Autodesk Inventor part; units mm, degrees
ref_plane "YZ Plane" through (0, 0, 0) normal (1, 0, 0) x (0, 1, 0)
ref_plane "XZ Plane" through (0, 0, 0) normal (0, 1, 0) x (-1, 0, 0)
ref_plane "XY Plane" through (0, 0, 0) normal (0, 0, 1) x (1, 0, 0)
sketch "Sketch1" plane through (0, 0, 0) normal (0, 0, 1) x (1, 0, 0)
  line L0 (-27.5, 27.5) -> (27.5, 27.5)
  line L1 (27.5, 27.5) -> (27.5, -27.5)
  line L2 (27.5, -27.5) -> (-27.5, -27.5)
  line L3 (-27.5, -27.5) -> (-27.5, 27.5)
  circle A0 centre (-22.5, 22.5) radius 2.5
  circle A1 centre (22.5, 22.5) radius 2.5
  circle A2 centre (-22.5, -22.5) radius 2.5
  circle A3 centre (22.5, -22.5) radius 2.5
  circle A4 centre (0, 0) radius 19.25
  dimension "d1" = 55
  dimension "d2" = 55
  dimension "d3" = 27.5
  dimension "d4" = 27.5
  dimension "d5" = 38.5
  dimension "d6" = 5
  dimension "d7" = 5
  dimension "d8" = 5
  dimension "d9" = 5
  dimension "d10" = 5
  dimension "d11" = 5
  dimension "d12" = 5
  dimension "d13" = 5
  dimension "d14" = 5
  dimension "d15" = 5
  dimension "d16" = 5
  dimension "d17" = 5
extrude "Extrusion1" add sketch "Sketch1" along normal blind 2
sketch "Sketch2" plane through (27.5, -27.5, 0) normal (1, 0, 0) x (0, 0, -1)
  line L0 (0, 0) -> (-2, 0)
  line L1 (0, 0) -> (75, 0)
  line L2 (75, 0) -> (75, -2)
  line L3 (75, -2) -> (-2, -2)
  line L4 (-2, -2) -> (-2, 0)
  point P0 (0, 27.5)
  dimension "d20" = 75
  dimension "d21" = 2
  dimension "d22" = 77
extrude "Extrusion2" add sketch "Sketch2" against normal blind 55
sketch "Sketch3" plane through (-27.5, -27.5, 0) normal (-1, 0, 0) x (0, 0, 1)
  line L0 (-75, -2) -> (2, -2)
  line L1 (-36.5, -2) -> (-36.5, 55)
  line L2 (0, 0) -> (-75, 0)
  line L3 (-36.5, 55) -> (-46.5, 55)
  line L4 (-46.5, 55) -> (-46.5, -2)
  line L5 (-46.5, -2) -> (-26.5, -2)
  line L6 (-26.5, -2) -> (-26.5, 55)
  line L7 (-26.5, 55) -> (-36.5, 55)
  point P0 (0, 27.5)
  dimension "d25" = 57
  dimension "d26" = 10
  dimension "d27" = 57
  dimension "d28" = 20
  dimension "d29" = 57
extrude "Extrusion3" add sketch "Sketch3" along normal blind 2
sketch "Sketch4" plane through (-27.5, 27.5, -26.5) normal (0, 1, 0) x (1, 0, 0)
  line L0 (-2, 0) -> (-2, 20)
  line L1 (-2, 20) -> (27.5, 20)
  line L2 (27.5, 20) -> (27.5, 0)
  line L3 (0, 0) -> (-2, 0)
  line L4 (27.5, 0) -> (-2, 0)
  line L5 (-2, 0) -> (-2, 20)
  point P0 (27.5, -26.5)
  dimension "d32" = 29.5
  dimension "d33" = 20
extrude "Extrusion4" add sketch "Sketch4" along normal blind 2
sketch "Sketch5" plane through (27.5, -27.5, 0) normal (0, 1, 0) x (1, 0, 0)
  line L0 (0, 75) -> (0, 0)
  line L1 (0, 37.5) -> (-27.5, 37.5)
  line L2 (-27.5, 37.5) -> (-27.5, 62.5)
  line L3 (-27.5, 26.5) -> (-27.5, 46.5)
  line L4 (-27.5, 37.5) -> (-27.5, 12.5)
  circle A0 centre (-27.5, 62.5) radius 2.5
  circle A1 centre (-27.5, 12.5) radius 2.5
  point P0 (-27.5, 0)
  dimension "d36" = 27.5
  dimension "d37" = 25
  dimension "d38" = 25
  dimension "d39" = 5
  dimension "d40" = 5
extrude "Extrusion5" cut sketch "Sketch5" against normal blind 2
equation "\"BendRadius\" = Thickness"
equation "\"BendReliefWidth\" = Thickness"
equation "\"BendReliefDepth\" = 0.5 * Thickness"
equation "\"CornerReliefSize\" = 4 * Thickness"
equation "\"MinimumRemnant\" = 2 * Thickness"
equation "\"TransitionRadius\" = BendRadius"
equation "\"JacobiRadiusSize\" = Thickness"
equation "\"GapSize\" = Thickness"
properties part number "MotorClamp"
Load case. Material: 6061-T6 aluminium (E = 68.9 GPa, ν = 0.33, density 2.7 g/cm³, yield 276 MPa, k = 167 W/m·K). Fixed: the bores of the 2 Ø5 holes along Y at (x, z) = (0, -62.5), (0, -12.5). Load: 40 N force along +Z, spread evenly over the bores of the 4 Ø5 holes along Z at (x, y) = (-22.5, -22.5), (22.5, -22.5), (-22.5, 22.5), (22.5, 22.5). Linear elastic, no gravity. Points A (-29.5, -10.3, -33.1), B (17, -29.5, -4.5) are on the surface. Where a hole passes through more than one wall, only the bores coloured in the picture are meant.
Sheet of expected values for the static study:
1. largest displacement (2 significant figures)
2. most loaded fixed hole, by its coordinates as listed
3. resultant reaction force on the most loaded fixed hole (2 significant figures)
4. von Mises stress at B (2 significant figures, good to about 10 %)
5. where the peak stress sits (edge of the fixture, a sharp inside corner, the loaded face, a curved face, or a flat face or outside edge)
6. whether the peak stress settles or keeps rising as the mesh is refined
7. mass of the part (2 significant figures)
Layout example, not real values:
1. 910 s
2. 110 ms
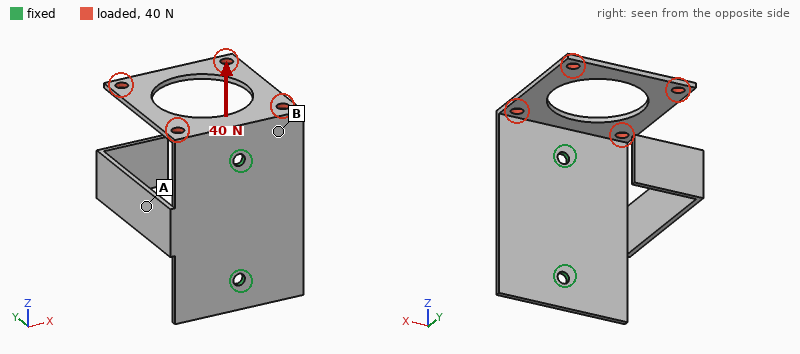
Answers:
1. 1.2 mm
2. (0, -12.5)
3. 26 N
4. 24 MPa
5. edge of the fixture
6. keeps rising
7. 42 g
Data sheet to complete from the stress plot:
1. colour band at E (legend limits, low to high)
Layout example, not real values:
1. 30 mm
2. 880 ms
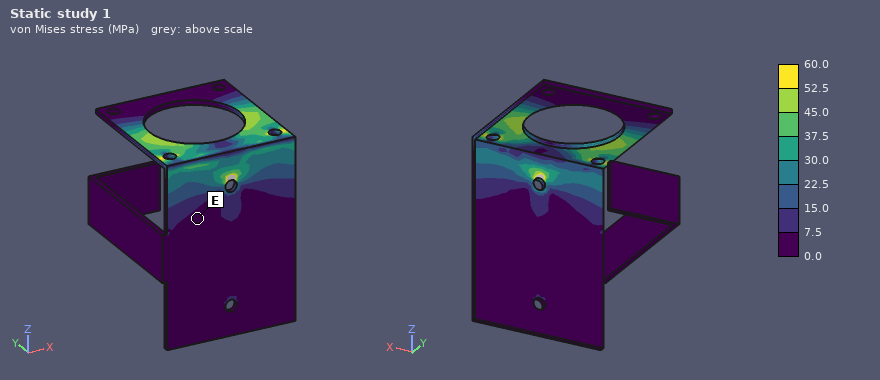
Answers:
1. 0.0 to 7.5 MPa
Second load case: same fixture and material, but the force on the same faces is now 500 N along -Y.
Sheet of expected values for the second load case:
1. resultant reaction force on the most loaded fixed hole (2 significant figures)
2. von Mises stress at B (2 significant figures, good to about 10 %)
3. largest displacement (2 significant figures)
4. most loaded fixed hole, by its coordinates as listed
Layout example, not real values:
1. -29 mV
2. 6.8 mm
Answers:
1. 540 N
2. 48 MPa
3. 1.2 mm
4. (0, -12.5)
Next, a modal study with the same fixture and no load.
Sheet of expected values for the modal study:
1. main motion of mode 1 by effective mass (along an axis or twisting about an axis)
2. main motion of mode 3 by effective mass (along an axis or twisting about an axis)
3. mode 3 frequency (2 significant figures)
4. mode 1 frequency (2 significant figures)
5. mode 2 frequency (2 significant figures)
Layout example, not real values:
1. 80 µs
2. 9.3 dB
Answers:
1. along X
2. along Z
3. 460 Hz
4. 220 Hz
5. 360 Hz
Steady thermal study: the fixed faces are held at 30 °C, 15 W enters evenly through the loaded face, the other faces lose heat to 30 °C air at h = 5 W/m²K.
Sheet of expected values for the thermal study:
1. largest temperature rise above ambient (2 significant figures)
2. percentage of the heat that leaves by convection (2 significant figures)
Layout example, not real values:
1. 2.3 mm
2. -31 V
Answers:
1. 71 K
2. 8.5 %
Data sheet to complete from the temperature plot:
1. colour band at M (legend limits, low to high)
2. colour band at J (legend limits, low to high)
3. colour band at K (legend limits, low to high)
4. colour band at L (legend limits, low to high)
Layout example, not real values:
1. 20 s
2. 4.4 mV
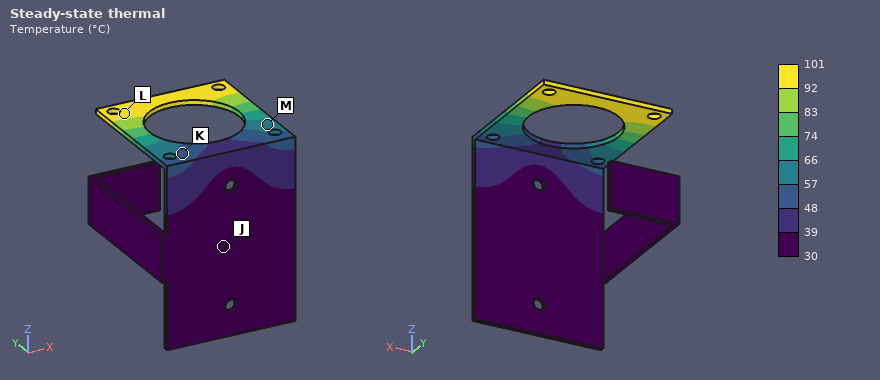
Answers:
1. 57 to 66 °C
2. 30 to 39 °C
3. 48 to 57 °C
4. 92 to 101 °C
